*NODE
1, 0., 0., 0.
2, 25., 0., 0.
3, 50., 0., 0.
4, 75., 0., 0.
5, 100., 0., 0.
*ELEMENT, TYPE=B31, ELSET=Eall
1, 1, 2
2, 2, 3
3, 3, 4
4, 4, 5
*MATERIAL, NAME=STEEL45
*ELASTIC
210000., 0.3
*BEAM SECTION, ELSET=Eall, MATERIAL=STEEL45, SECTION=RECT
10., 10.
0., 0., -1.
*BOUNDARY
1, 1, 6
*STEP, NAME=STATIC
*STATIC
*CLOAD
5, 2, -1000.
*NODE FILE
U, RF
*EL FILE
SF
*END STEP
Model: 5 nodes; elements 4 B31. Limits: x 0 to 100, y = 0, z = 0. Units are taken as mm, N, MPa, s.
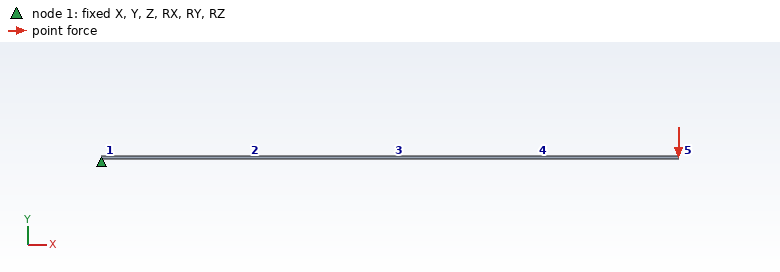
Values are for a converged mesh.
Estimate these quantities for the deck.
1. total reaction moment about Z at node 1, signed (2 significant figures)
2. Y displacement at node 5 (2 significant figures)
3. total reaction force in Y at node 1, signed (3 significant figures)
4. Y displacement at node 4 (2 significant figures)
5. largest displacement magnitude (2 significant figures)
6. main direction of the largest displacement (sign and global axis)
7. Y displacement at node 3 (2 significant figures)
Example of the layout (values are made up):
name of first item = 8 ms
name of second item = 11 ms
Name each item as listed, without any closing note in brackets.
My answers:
total reaction moment about Z at node 1, signed = 1.0e+05 N·mm
Y displacement at node 5 = -1.9 mm
total reaction force in Y at node 1, signed = 1000 N
Y displacement at node 4 = -1.2 mm
largest displacement magnitude = 1.9 mm
main direction of the largest displacement = -Y
Y displacement at node 3 = -0.60 mm
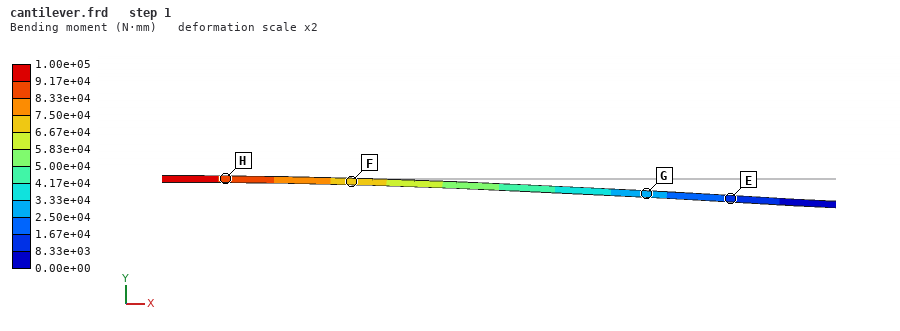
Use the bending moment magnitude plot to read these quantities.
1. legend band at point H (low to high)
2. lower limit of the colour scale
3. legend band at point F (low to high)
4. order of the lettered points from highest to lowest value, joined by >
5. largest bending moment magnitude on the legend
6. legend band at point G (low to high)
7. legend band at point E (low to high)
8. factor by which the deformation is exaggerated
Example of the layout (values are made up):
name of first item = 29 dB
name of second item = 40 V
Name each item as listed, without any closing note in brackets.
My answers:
legend band at point H = 8.33e+04 to 9.17e+04 N·mm
lower limit of the colour scale = 0.00e+00 N·mm
legend band at point F = 6.67e+04 to 7.50e+04 N·mm
order of the lettered points from highest to lowest value, joined by > = H > F > G > E
largest bending moment magnitude on the legend = 1.00e+05 N·mm
legend band at point G = 2.50e+04 to 3.33e+04 N·mm
legend band at point E = 8.33e+03 to 1.67e+04 N·mm
factor by which the deformation is exaggerated = 2
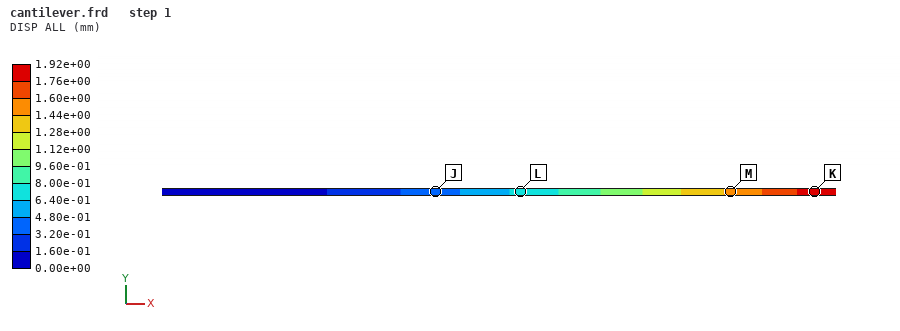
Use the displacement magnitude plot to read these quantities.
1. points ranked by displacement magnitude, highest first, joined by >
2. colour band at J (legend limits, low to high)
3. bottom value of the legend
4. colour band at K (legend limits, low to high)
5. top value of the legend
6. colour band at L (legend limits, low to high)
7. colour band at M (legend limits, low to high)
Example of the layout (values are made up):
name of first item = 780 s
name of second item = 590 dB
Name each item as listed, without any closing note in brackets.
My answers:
points ranked by displacement magnitude, highest first, joined by > = K > M > L > J
colour band at J = 3.20e-01 to 4.80e-01 mm
bottom value of the legend = 0.00e+00 mm
colour band at K = 1.76e+00 to 1.92e+00 mm
top value of the legend = 1.92e+00 mm
colour band at L = 6.40e-01 to 8.00e-01 mm
colour band at M = 1.44e+00 to 1.60e+00 mm
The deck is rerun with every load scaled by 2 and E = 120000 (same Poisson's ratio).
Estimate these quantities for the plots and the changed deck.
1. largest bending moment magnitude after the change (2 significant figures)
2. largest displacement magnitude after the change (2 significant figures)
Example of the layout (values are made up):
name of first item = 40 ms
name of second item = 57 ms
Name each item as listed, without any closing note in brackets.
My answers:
largest bending moment magnitude after the change = 2.0e+05 N·mm
largest displacement magnitude after the change = 6.7 mm
